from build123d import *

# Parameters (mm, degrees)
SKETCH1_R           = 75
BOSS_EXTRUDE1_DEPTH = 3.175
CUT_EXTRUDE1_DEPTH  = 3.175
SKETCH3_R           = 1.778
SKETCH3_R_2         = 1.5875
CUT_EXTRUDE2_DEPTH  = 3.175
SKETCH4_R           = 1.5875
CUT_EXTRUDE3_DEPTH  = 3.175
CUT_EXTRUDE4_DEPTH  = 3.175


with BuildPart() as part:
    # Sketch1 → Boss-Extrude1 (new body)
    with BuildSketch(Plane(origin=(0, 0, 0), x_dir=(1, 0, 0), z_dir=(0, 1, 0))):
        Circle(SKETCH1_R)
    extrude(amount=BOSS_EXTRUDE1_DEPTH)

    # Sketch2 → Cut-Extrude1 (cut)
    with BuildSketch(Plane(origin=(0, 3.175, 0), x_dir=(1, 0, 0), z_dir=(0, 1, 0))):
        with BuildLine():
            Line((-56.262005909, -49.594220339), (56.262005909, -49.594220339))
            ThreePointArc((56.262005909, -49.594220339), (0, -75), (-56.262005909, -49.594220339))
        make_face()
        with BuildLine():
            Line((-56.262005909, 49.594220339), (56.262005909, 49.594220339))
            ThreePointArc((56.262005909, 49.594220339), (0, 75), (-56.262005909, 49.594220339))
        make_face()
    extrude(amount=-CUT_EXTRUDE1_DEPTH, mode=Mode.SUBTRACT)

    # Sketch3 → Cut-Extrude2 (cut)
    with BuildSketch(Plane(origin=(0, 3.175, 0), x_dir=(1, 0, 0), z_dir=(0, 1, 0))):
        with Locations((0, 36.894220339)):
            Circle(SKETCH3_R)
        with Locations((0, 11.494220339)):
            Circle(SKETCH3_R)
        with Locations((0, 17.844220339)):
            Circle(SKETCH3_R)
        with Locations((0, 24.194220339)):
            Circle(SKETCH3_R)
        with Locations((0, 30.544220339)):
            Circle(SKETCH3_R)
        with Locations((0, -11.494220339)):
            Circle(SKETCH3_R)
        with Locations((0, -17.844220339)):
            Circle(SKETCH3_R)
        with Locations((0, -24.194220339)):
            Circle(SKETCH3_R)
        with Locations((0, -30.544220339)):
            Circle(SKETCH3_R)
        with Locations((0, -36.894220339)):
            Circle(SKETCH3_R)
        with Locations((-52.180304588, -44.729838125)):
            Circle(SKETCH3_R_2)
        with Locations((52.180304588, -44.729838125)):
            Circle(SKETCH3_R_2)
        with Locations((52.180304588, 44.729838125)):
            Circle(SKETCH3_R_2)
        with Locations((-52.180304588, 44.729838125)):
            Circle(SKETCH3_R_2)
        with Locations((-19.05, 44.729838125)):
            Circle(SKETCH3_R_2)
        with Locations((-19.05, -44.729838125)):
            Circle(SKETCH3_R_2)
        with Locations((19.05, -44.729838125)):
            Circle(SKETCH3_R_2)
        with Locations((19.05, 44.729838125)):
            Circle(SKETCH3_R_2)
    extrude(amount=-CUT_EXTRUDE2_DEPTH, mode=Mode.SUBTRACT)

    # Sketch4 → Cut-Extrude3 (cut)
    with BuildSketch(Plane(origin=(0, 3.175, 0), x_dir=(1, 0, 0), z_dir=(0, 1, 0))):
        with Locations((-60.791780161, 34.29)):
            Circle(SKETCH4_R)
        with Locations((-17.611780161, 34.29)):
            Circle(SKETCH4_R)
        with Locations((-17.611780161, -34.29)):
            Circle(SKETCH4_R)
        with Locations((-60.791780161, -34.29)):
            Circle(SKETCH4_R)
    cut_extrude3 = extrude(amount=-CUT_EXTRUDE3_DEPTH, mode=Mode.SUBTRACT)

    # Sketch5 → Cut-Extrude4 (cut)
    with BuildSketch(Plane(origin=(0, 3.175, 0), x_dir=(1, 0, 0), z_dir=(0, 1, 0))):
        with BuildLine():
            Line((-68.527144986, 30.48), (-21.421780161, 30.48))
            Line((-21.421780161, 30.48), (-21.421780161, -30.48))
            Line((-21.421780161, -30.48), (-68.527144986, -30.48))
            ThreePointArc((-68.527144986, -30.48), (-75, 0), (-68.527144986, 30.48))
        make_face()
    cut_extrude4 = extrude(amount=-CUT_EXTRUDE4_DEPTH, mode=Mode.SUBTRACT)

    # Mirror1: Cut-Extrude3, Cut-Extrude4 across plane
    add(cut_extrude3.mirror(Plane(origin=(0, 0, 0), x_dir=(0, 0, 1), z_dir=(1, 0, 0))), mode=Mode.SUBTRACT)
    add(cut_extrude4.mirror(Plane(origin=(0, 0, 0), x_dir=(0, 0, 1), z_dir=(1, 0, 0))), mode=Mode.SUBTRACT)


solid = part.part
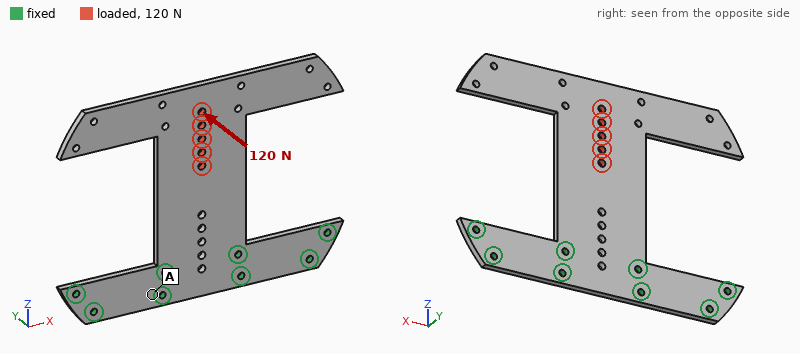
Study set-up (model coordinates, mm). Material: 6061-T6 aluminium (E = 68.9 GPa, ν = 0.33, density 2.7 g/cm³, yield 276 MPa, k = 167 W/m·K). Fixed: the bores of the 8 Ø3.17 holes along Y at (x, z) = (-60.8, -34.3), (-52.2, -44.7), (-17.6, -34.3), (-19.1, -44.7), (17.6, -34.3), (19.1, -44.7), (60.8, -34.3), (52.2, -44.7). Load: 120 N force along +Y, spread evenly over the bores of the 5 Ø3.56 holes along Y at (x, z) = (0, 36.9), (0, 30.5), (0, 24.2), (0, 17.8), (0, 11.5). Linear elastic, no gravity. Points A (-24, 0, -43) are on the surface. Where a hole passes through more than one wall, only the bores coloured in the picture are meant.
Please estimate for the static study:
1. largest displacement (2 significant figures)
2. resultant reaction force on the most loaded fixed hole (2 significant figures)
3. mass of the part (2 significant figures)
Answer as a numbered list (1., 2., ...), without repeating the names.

1. 1.9 mm
2. 200 N
3. 62 g
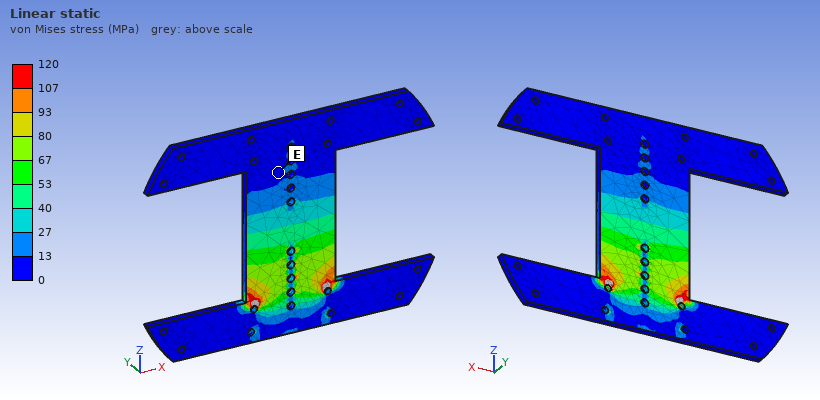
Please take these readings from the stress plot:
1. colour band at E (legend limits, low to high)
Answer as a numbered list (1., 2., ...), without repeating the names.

1. 0 to 13 MPa
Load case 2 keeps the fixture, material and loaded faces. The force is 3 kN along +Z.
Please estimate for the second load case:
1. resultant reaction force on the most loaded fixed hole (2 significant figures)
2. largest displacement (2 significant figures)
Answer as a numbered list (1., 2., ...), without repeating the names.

1. 1.2 kN
2. 26 µm
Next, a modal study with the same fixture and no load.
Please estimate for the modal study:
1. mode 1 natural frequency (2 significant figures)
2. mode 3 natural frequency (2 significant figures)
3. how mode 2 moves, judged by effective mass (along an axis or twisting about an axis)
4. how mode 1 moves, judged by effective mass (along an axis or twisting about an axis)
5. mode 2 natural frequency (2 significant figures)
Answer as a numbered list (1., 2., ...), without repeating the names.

1. 240 Hz
2. 1100 Hz
3. twisting about Z
4. along Y
5. 390 Hz
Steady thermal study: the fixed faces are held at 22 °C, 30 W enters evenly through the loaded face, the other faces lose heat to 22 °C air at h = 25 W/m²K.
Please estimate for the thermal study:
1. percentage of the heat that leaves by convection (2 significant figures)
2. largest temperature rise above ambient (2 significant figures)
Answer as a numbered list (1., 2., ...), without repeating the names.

1. 38 %
2. 59 K
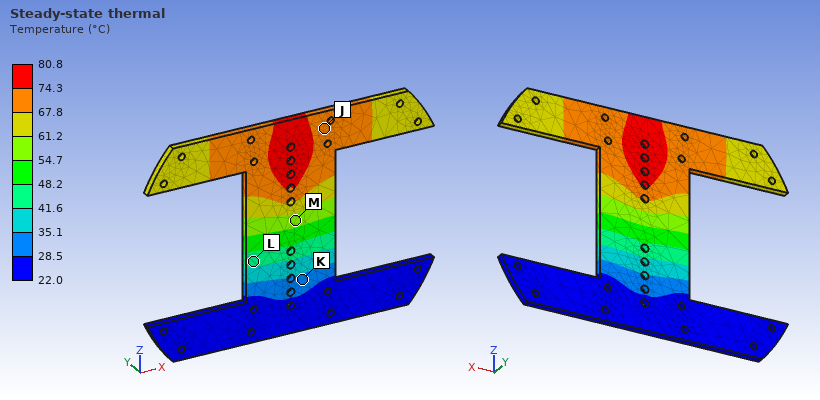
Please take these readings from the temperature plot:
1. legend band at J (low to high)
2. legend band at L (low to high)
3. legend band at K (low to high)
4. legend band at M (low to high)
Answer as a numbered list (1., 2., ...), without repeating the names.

1. 67.8 to 74.3 °C
2. 41.6 to 48.2 °C
3. 28.5 to 35.1 °C
4. 54.7 to 61.2 °C
